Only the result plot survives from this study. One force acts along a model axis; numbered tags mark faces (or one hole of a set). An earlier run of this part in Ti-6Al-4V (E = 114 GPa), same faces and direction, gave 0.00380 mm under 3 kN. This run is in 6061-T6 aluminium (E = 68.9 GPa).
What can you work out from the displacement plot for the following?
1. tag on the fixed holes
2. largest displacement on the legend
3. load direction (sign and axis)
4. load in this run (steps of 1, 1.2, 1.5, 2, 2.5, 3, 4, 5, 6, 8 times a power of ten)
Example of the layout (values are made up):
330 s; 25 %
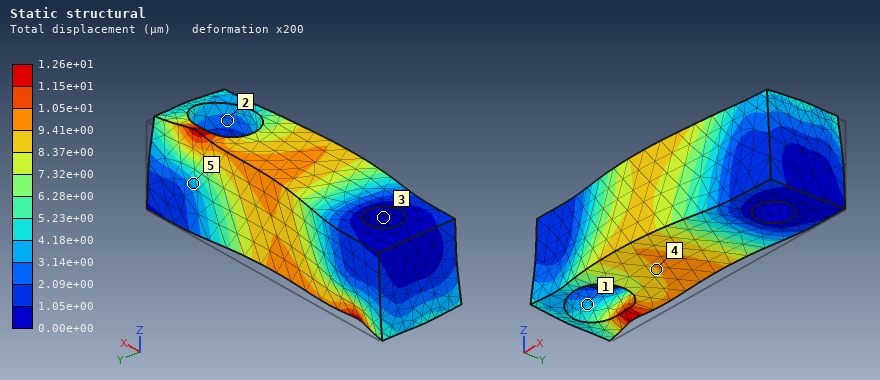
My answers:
3; 1.26e+01 µm; -Y; 6 kN
